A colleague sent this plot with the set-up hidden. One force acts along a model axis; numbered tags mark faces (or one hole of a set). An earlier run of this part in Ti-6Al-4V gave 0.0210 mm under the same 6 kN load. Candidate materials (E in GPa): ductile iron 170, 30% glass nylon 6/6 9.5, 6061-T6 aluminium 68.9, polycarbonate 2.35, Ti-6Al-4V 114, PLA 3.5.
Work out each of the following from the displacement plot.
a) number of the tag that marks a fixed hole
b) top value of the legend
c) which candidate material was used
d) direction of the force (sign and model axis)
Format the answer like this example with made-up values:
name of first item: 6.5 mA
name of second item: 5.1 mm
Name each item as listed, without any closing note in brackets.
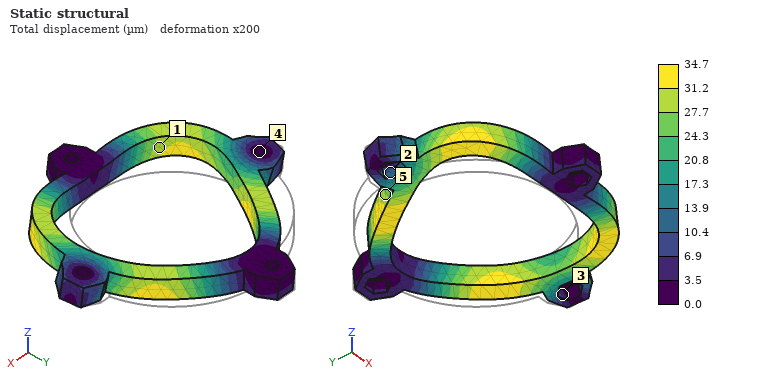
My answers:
number of the tag that marks a fixed hole: 4
top value of the legend: 34.7 µm
which candidate material was used: 6061-T6 aluminium
direction of the force: -Y
